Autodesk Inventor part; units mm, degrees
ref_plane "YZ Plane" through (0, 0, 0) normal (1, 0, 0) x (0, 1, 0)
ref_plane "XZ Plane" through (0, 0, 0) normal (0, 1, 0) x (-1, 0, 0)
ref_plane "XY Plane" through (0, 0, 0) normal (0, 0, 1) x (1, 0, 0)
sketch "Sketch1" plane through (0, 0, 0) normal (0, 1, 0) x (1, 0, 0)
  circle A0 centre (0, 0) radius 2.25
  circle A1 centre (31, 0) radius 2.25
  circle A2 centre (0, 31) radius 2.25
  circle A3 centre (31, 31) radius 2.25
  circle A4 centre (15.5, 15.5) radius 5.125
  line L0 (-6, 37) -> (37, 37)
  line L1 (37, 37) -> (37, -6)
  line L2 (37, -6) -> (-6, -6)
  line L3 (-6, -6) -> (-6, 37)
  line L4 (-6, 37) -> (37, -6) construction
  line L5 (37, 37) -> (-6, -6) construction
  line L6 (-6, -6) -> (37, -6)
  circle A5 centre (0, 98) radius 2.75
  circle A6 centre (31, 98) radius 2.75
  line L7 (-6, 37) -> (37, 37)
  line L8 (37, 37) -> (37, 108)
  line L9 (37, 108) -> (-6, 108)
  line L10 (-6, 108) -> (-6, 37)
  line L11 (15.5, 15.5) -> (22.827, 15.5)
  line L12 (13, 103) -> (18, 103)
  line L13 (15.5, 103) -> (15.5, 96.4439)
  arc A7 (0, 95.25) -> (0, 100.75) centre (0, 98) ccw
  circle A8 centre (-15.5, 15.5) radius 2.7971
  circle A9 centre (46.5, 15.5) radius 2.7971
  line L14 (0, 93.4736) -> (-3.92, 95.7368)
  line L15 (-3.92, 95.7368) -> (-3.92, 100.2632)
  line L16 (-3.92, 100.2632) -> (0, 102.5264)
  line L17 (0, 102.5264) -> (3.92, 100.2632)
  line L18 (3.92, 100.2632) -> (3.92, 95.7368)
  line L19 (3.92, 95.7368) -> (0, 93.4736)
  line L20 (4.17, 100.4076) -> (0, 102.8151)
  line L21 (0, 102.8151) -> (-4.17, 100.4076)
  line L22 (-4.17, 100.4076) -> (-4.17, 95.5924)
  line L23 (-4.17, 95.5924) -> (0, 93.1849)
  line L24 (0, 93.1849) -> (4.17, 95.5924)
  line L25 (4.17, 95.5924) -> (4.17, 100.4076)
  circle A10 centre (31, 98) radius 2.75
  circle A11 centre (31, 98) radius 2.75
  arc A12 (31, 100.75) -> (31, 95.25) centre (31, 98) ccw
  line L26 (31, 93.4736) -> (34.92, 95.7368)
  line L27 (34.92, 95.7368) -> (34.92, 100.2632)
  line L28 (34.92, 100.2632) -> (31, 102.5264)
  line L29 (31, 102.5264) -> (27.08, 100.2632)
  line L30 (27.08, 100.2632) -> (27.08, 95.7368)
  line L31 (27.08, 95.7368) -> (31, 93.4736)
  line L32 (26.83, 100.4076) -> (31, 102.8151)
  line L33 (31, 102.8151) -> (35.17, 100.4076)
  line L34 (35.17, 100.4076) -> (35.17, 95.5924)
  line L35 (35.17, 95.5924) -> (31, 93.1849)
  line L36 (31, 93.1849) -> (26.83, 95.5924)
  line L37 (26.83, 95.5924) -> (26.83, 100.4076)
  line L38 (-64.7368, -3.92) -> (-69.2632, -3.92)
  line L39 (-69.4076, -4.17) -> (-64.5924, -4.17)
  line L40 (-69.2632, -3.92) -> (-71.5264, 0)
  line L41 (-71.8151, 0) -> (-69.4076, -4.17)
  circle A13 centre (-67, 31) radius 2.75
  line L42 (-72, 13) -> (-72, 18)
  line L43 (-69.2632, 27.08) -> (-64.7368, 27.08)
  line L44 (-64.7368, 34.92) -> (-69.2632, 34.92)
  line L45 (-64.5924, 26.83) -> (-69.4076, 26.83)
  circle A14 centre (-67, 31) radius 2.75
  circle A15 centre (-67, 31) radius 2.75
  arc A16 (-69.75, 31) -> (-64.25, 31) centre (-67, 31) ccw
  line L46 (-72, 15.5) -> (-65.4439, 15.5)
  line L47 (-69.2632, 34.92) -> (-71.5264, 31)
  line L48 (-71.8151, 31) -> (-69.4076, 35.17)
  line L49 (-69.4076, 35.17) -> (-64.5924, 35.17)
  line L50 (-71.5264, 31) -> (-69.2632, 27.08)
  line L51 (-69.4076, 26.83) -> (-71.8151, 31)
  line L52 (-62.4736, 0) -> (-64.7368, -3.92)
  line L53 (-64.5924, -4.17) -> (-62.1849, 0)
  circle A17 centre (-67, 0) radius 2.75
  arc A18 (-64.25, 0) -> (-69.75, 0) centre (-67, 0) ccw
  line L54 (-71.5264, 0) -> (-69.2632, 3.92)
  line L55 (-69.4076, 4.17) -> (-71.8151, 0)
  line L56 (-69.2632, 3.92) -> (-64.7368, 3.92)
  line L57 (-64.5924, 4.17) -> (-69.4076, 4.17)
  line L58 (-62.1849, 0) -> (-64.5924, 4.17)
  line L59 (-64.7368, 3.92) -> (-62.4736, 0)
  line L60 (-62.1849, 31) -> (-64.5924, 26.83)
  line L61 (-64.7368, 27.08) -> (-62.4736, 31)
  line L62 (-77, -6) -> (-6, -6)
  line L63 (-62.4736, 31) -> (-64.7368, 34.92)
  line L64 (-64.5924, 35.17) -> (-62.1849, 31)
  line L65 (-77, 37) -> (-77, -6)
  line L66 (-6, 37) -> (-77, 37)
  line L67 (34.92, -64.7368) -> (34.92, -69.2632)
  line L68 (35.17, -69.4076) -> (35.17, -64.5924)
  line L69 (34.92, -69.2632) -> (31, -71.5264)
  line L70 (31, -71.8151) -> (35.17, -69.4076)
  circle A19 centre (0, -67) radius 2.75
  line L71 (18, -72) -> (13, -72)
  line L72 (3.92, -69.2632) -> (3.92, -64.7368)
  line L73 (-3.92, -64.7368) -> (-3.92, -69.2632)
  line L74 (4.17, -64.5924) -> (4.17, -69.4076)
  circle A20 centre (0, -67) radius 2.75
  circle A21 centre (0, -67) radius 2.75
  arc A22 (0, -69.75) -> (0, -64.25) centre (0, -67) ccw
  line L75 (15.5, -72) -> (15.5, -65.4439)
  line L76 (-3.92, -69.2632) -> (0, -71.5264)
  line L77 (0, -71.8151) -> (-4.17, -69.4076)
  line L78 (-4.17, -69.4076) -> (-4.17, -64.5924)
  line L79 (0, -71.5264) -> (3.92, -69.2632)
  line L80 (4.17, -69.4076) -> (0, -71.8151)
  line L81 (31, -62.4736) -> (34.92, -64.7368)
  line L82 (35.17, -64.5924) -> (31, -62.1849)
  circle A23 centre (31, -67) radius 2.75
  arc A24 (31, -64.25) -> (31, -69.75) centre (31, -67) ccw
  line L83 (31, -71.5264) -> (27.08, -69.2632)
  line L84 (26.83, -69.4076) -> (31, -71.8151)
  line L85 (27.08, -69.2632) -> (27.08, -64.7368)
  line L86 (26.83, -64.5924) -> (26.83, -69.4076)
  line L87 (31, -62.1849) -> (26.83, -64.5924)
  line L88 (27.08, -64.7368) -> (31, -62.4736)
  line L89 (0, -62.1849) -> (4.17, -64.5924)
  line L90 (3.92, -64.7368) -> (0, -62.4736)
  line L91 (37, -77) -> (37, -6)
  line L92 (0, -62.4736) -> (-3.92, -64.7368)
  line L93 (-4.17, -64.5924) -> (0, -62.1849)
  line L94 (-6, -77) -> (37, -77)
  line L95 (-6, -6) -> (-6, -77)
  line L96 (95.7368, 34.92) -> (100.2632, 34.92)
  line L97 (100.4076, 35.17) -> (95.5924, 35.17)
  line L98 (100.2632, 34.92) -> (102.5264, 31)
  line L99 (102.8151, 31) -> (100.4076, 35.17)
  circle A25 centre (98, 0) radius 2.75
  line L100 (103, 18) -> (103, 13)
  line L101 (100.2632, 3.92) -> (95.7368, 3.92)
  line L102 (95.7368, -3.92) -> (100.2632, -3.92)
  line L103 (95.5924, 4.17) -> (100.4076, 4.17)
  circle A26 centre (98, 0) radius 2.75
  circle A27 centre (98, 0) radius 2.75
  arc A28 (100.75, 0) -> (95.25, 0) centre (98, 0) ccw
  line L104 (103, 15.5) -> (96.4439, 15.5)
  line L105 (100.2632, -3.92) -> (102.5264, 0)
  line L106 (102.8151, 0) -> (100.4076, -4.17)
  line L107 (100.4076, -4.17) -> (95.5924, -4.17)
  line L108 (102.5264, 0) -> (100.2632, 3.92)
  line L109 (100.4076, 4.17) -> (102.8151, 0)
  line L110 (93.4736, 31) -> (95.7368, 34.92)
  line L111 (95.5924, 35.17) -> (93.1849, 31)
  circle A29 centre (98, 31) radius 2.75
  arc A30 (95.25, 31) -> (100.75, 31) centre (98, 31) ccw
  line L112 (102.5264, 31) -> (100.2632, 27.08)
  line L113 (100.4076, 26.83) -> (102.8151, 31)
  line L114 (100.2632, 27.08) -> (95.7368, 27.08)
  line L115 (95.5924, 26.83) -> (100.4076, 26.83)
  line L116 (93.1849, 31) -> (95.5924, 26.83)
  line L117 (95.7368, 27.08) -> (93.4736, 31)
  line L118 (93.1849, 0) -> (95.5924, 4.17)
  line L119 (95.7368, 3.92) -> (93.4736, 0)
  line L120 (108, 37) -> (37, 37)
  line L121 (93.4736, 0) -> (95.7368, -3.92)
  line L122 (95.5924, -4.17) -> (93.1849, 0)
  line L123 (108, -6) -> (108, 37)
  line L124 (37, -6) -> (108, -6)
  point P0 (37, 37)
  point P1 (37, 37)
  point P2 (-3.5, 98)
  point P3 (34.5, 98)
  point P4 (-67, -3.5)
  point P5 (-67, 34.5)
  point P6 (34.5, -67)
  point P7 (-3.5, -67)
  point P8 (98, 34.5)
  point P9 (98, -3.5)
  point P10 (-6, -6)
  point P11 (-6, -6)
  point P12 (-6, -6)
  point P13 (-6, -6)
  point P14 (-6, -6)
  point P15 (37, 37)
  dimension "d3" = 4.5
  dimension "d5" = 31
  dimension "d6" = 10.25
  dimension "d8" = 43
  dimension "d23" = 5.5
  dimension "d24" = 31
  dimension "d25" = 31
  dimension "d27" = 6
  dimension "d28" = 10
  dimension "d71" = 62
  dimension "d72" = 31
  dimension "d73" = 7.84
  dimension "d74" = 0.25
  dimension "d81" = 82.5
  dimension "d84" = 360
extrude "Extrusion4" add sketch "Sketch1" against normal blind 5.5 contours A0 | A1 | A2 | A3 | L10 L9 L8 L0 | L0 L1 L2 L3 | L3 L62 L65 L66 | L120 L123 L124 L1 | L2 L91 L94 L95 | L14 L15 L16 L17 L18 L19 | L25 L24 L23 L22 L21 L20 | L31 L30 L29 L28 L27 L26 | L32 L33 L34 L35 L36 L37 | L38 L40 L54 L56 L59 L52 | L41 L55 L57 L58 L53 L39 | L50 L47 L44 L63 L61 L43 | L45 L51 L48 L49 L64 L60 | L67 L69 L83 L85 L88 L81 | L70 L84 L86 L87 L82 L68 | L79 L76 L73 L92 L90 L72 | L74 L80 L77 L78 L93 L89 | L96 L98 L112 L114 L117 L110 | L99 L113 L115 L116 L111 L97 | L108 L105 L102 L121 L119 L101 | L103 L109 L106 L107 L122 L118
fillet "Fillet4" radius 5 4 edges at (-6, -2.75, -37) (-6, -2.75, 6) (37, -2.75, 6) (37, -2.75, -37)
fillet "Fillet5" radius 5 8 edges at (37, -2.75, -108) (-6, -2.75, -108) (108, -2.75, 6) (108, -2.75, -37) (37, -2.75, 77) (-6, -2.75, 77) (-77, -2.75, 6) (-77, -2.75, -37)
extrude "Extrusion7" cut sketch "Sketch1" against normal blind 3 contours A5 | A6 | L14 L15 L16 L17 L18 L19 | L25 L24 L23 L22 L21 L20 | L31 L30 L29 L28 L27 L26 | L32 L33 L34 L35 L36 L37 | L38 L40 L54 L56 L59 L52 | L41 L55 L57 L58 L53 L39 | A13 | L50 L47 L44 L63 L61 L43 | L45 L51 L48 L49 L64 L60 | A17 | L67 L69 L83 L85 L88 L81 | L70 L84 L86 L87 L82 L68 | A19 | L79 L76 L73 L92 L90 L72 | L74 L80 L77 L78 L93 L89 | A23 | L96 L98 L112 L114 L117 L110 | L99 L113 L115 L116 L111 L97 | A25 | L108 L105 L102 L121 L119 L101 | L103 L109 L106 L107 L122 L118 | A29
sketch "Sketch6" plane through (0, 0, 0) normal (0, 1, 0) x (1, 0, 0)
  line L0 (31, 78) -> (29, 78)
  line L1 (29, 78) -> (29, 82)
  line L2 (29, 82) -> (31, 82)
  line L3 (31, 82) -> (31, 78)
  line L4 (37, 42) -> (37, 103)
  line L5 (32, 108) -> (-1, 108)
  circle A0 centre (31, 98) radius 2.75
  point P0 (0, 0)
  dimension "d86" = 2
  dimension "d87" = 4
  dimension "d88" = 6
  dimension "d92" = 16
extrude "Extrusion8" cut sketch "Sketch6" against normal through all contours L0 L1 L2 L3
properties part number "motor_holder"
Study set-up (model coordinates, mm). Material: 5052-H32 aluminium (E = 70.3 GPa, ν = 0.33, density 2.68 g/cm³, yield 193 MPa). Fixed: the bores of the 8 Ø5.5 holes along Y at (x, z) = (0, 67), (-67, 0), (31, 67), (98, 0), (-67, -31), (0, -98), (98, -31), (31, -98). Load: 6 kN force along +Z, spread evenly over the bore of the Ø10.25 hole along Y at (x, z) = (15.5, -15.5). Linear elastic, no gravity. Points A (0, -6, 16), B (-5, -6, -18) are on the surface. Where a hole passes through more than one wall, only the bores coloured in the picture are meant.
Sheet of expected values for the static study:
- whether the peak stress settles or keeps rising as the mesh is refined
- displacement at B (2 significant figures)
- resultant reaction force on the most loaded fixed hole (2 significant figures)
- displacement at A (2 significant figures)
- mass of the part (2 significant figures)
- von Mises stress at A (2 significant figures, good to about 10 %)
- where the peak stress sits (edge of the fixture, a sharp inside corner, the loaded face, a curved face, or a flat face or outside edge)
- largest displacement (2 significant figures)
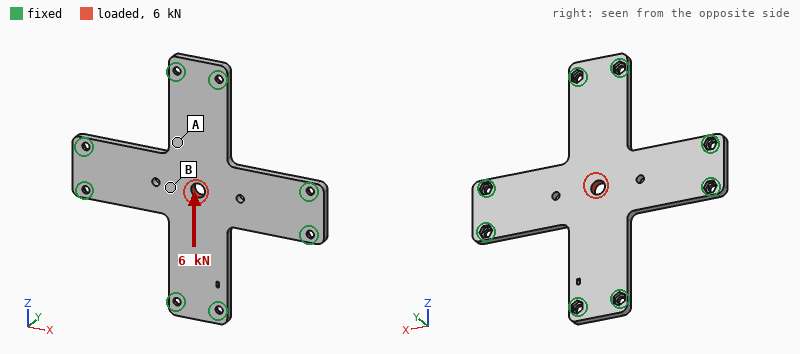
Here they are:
keeps rising
13 µm
1.3 kN
15 µm
200 g
12 MPa
edge of the fixture
20 µm
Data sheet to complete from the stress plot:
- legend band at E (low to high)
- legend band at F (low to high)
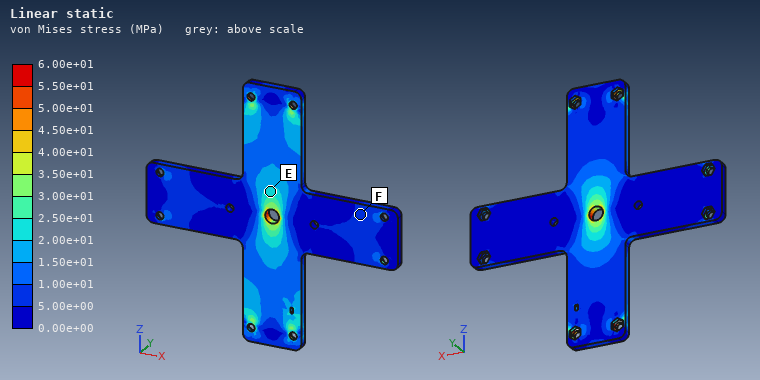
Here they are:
2.00e+01 to 2.50e+01 MPa
5.00e+00 to 1.00e+01 MPa
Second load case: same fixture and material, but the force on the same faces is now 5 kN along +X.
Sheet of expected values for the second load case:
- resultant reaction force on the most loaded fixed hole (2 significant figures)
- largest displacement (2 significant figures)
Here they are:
1.1 kN
17 µm
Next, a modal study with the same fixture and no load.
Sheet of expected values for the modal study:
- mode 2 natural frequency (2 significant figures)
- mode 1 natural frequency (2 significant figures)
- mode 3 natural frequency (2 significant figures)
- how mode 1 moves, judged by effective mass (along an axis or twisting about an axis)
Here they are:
2700 Hz
1200 Hz
2800 Hz
along Y
